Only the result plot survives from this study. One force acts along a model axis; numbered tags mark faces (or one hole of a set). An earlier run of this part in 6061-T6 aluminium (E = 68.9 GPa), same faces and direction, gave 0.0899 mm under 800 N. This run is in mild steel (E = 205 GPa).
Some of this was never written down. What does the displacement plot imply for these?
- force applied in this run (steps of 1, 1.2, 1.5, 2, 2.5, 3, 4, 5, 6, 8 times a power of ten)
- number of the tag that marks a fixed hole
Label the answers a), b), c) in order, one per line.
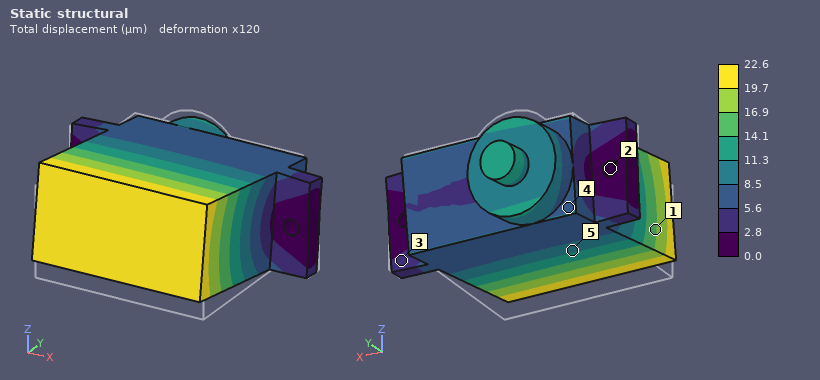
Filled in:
a) 600 N
b) 2
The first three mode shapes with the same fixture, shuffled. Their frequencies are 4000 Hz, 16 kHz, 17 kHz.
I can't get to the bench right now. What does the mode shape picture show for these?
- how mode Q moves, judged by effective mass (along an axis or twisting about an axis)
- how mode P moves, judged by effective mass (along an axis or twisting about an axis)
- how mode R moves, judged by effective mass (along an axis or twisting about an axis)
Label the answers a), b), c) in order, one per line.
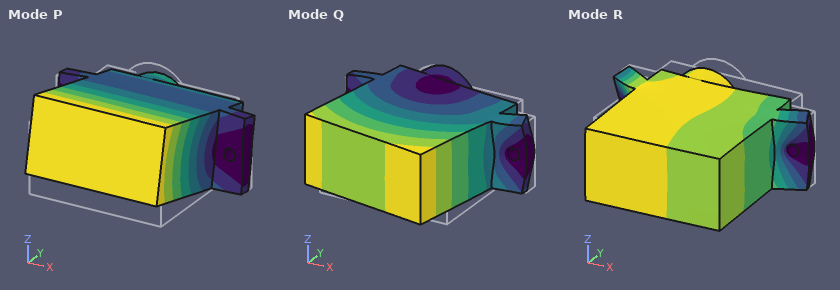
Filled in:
a) along X
b) along Z
c) along Y
